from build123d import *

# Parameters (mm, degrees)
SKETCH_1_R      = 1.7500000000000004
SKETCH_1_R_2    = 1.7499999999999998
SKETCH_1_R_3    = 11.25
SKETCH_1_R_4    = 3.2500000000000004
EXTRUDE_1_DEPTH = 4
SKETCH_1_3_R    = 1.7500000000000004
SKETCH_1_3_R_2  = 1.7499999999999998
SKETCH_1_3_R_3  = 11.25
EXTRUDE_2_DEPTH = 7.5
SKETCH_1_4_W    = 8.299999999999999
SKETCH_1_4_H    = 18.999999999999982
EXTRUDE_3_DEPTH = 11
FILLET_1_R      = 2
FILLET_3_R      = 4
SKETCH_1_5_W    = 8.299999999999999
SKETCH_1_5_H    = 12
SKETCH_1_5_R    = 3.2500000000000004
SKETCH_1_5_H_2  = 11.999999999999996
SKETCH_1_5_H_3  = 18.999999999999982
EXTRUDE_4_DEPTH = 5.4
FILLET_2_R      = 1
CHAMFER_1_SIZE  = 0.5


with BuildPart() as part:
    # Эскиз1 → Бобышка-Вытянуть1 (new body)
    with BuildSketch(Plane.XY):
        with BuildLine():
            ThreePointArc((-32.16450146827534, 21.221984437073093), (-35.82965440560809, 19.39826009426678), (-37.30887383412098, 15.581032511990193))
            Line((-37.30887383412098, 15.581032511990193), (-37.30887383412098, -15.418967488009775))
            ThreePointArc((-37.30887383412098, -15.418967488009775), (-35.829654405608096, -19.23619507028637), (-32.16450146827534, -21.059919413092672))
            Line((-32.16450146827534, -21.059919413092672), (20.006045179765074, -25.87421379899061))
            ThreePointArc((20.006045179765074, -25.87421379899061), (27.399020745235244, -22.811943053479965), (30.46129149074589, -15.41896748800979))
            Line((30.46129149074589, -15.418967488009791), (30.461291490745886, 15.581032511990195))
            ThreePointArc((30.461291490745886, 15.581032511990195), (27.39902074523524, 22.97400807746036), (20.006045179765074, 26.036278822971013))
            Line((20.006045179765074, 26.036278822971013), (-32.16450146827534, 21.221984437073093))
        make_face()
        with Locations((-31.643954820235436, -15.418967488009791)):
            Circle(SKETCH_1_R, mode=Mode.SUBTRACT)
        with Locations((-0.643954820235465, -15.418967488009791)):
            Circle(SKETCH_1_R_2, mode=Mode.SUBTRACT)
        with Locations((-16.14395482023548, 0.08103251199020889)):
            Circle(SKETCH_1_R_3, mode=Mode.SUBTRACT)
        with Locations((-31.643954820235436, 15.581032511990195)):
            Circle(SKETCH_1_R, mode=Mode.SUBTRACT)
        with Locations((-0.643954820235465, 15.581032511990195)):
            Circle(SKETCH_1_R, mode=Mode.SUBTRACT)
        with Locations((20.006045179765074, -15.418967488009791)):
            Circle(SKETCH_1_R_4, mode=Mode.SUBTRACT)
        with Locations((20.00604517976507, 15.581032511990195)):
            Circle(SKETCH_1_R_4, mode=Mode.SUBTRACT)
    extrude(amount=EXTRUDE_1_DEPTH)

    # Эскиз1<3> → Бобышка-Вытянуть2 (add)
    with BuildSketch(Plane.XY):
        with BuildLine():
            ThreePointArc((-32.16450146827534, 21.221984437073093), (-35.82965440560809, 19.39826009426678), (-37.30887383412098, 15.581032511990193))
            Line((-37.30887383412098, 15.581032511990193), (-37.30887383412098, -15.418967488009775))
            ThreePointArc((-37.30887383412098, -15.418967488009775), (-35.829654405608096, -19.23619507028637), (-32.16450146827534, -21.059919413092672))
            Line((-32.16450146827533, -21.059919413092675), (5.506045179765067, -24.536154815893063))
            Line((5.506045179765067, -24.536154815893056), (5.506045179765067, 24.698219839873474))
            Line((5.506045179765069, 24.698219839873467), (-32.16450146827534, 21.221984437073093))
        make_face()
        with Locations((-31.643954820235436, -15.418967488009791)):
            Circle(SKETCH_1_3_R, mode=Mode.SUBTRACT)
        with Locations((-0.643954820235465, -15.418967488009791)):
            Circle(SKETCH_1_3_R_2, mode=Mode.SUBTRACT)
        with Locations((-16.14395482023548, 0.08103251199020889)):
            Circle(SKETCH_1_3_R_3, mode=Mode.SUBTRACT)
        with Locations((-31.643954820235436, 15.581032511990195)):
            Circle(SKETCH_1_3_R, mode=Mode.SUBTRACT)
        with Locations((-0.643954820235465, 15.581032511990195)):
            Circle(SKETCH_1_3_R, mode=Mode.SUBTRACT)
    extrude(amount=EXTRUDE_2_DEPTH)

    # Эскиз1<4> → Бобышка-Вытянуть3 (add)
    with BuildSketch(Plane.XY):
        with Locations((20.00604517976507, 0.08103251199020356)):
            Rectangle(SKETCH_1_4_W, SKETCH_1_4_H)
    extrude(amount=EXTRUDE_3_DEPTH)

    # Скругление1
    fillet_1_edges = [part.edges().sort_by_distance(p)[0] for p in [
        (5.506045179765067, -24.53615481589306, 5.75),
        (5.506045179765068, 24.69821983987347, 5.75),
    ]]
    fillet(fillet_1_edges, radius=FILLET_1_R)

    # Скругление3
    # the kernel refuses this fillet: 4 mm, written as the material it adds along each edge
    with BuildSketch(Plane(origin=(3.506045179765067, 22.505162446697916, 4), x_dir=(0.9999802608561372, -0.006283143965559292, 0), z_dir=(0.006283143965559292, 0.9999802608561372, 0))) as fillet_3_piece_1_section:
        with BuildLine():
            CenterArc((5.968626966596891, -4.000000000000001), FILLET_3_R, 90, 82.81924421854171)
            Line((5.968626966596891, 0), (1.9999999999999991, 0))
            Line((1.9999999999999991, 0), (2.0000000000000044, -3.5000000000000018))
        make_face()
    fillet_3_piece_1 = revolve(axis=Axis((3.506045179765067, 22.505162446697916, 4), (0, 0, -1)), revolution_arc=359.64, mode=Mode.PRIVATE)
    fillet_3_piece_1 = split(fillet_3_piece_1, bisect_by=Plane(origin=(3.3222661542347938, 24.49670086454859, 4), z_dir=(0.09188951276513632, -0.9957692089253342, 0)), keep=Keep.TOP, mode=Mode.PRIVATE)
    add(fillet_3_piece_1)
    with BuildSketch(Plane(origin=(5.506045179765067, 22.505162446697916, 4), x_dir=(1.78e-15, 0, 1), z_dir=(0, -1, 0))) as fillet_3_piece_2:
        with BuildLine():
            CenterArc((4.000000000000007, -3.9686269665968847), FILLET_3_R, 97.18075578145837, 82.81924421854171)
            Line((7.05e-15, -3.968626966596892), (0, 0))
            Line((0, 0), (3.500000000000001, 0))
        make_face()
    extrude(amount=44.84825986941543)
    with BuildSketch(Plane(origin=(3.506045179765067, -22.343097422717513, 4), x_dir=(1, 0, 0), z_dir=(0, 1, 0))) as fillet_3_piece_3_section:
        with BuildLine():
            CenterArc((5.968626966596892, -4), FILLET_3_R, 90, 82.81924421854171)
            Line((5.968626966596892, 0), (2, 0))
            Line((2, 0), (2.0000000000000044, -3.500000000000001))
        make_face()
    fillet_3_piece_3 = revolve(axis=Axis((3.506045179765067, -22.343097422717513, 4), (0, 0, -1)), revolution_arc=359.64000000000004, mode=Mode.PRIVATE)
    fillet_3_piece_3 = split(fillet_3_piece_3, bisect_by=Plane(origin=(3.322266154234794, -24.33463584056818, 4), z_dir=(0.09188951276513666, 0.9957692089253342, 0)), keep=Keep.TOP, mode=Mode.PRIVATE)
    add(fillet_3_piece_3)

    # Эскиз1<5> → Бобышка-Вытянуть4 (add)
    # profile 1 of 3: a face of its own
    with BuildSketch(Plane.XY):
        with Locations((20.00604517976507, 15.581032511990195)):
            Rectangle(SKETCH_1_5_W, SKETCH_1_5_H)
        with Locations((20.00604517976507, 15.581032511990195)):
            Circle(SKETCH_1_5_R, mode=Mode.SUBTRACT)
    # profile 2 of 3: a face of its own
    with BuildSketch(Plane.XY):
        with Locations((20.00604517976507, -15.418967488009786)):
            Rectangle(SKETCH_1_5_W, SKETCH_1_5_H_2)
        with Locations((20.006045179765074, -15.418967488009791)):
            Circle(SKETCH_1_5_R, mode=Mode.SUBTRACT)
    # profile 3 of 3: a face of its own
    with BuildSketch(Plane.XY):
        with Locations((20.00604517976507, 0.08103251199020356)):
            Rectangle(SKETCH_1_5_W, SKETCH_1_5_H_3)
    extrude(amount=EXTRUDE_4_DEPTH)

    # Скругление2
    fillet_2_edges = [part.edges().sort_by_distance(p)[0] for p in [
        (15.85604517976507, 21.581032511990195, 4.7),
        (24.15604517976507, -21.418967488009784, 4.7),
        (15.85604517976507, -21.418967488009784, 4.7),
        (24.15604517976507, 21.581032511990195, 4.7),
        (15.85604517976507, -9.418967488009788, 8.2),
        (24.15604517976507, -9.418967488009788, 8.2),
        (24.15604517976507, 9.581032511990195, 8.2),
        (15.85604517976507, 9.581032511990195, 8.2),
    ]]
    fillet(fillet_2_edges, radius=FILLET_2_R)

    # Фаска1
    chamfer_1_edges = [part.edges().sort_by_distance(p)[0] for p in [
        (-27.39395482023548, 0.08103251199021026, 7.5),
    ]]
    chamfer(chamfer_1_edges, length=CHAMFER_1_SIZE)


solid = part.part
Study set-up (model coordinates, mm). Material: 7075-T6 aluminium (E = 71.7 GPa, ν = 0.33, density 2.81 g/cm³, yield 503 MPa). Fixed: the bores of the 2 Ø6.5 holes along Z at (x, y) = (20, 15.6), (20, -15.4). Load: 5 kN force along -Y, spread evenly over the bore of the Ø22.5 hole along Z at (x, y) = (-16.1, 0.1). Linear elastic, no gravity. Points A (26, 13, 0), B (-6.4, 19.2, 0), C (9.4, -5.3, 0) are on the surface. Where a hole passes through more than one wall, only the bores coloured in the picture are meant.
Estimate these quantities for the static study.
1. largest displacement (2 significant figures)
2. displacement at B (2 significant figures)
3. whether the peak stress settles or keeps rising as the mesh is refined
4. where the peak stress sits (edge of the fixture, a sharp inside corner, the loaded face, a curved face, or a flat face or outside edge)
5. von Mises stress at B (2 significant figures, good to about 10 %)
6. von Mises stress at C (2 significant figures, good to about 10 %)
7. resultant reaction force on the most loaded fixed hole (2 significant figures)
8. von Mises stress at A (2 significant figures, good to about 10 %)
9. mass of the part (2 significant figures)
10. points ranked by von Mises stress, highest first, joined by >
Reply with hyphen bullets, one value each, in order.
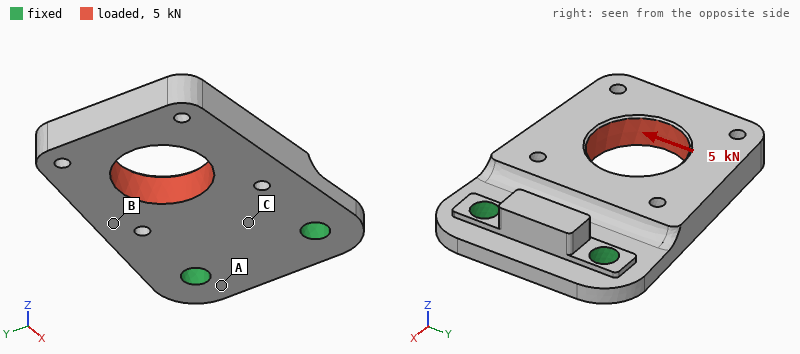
- 0.12 mm
- 0.052 mm
- keeps rising
- edge of the fixture
- 44 MPa
- 71 MPa
- 5.6 kN
- 20 MPa
- 49 g
- C > B > A
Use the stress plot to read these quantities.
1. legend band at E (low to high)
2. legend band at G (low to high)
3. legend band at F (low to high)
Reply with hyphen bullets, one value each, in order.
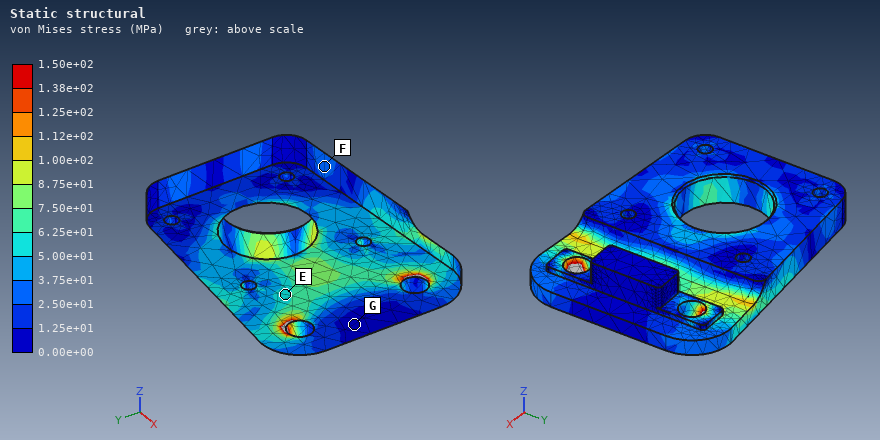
- 5.00e+01 to 6.25e+01 MPa
- 0.00e+00 to 1.25e+01 MPa
- 2.50e+01 to 3.75e+01 MPa
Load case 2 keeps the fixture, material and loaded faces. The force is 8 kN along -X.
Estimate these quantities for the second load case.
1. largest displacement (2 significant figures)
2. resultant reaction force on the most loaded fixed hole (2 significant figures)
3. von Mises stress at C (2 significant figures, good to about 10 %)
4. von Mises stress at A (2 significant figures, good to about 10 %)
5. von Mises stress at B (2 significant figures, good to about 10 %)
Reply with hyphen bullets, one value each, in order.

- 0.31 mm
- 4.0 kN
- 46 MPa
- 16 MPa
- 36 MPa
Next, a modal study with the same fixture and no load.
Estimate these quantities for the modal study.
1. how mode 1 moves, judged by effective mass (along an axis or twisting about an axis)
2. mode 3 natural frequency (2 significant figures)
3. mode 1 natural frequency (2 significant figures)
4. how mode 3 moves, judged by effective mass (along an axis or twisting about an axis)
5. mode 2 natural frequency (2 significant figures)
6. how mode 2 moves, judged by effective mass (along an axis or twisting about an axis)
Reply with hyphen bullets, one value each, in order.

- along Z
- 7000 Hz
- 1100 Hz
- along Y
- 4000 Hz
- twisting about X
